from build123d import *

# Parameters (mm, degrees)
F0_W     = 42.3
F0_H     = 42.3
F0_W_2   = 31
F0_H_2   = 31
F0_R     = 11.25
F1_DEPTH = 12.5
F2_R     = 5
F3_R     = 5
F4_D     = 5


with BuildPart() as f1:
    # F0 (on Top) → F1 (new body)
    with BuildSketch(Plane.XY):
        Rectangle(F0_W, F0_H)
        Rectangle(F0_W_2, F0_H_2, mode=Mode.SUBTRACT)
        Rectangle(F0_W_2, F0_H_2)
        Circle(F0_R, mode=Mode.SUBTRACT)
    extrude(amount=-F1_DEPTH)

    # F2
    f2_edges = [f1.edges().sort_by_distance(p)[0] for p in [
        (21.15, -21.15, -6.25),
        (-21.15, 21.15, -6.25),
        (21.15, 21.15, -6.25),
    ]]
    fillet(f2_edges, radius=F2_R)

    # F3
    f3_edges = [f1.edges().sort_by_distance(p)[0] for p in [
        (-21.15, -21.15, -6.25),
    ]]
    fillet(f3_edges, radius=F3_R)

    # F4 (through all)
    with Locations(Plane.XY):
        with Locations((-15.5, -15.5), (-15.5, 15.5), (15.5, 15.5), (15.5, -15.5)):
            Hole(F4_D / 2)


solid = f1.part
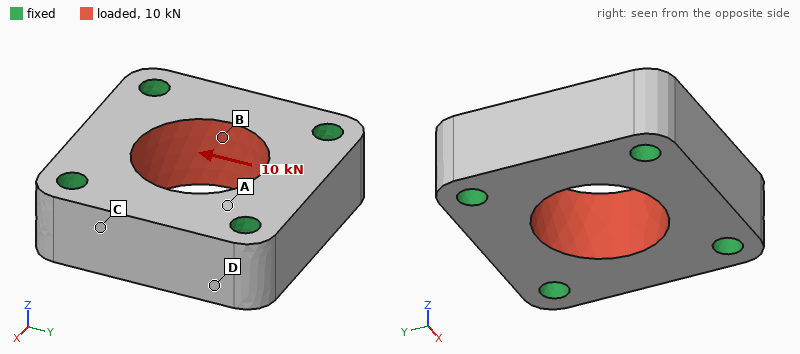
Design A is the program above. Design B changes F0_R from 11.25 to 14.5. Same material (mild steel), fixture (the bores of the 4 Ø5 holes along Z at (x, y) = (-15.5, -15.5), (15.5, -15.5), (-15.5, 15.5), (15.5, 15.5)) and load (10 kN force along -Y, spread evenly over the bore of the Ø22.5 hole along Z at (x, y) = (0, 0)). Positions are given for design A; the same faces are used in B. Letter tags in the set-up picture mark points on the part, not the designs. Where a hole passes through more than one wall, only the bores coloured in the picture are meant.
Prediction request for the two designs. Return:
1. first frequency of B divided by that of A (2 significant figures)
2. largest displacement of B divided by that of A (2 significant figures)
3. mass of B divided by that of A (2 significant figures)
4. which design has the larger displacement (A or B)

1.1
1.3
0.80
B
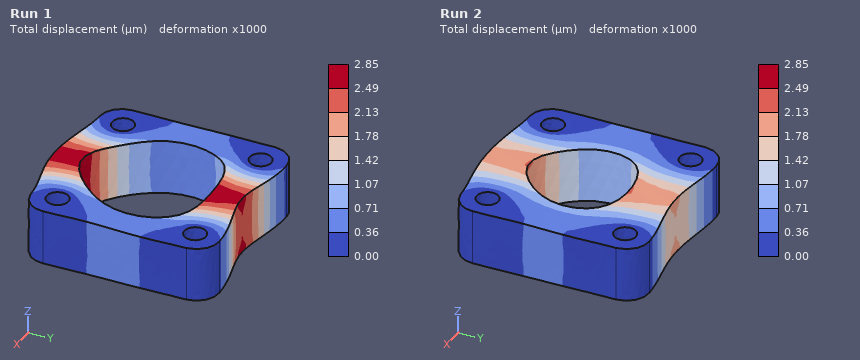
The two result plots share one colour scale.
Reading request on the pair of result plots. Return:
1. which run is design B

Run 1
